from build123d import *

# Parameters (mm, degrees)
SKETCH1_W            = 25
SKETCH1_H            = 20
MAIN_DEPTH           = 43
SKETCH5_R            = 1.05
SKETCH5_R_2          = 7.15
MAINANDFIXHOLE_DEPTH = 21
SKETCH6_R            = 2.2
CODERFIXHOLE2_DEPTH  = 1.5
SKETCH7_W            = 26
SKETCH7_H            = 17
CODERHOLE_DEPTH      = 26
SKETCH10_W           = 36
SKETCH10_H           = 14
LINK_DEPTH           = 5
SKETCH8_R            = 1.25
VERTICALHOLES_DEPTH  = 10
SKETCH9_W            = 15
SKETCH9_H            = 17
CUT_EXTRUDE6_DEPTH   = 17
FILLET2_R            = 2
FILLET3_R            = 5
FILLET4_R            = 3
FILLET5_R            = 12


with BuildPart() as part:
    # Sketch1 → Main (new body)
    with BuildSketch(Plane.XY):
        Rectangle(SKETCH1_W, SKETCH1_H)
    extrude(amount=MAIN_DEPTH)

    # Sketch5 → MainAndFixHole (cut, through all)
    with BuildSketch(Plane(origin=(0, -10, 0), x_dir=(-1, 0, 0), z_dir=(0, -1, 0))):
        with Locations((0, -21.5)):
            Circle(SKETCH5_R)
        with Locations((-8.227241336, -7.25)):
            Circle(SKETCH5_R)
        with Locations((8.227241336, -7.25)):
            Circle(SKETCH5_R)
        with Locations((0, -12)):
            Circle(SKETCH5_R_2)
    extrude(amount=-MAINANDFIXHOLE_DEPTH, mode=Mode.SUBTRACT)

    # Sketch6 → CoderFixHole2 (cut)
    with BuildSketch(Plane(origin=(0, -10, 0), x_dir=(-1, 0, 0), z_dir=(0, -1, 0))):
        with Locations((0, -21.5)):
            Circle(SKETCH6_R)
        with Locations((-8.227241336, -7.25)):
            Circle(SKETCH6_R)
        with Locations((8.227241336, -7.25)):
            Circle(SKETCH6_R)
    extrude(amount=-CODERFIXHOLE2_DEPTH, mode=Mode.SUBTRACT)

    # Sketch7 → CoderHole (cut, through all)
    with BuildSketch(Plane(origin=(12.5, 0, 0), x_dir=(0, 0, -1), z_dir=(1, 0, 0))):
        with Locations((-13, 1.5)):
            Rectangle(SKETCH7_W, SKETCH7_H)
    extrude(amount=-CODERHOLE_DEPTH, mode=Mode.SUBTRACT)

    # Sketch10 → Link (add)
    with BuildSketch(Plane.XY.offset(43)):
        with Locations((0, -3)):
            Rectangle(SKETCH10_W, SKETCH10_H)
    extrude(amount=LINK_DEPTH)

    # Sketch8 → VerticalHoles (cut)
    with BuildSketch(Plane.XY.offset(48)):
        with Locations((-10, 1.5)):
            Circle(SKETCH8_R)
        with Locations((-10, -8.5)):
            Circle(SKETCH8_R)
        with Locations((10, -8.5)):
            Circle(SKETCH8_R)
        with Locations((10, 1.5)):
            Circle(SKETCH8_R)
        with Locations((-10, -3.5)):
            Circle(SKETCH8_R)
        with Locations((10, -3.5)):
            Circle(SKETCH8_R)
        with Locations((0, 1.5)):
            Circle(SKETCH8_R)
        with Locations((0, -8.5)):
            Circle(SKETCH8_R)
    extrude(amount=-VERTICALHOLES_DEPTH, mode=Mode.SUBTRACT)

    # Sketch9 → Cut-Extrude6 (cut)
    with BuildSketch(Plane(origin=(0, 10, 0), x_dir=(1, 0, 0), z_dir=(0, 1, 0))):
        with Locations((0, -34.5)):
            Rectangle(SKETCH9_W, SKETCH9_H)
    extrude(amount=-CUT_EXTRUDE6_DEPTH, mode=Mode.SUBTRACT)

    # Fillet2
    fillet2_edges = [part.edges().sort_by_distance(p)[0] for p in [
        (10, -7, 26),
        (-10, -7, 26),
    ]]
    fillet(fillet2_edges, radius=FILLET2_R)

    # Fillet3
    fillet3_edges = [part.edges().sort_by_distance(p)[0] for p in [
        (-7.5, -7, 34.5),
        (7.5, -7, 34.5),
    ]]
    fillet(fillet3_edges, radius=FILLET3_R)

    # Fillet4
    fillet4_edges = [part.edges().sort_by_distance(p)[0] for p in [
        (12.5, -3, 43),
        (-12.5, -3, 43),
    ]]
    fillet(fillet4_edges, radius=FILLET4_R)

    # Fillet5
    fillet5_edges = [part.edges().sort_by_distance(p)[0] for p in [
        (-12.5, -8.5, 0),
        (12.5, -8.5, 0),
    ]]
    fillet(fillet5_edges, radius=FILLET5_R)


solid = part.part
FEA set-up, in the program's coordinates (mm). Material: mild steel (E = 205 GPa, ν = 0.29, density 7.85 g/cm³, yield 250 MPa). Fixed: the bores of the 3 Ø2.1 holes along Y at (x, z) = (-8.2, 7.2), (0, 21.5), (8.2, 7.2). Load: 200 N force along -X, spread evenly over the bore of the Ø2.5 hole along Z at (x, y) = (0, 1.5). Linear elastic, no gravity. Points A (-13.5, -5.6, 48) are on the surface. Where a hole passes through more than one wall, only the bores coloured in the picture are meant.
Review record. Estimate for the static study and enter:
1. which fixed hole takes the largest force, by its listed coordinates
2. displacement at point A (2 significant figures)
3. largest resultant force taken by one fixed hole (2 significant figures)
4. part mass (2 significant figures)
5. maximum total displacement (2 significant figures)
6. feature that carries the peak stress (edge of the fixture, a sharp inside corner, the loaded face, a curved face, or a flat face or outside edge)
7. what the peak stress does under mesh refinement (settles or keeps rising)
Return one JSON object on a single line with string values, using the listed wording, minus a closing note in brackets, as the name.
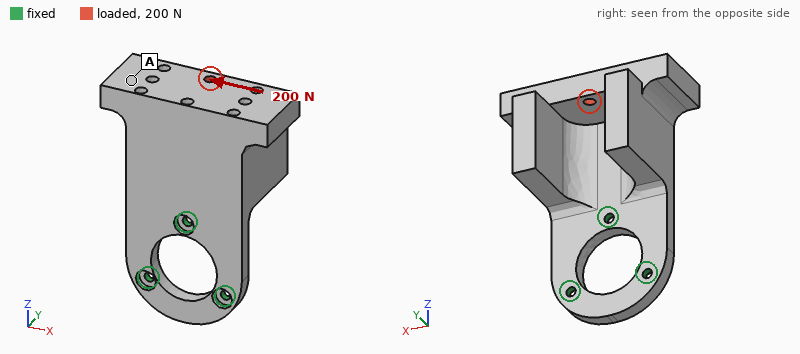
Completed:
{"which fixed hole takes the largest force, by its listed coordinates": "(0, 21.5)", "displacement at point A": "27 µm", "largest resultant force taken by one fixed hole": "310 N", "part mass": "61 g", "maximum total displacement": "43 µm", "feature that carries the peak stress": "edge of the fixture", "what the peak stress does under mesh refinement": "keeps rising"}
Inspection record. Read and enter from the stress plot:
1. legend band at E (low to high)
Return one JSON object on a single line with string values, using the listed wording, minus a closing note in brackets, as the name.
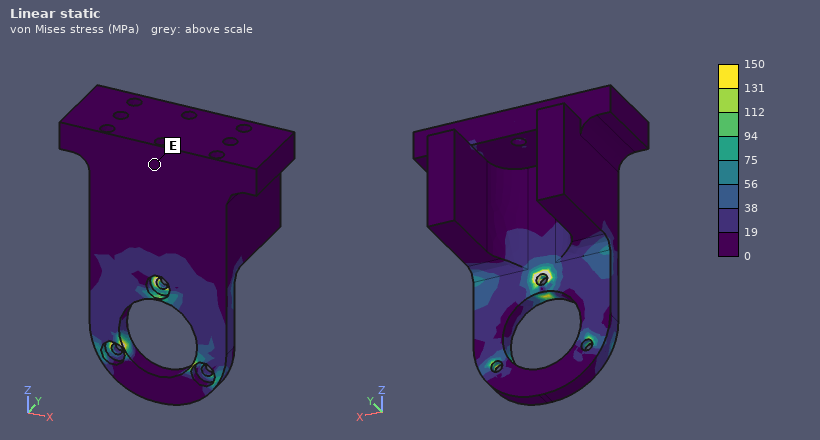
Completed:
{"legend band at E": "0 to 19 MPa"}
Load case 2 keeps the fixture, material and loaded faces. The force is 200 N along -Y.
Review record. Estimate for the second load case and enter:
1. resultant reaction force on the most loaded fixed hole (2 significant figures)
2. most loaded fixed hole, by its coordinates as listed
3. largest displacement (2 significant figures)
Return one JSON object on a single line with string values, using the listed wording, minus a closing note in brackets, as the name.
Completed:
{"resultant reaction force on the most loaded fixed hole": "590 N", "most loaded fixed hole, by its coordinates as listed": "(0, 21.5)", "largest displacement": "0.11 mm"}
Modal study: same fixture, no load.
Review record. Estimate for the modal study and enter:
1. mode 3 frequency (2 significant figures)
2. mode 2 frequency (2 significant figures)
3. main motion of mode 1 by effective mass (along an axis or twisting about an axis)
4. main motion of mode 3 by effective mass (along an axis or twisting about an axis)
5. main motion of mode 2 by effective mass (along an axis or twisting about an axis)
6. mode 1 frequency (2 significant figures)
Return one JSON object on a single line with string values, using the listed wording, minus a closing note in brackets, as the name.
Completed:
{"mode 3 frequency": "5700 Hz", "mode 2 frequency": "1800 Hz", "main motion of mode 1 by effective mass": "along Y", "main motion of mode 3 by effective mass": "along X", "main motion of mode 2 by effective mass": "along X", "mode 1 frequency": "1300 Hz"}
